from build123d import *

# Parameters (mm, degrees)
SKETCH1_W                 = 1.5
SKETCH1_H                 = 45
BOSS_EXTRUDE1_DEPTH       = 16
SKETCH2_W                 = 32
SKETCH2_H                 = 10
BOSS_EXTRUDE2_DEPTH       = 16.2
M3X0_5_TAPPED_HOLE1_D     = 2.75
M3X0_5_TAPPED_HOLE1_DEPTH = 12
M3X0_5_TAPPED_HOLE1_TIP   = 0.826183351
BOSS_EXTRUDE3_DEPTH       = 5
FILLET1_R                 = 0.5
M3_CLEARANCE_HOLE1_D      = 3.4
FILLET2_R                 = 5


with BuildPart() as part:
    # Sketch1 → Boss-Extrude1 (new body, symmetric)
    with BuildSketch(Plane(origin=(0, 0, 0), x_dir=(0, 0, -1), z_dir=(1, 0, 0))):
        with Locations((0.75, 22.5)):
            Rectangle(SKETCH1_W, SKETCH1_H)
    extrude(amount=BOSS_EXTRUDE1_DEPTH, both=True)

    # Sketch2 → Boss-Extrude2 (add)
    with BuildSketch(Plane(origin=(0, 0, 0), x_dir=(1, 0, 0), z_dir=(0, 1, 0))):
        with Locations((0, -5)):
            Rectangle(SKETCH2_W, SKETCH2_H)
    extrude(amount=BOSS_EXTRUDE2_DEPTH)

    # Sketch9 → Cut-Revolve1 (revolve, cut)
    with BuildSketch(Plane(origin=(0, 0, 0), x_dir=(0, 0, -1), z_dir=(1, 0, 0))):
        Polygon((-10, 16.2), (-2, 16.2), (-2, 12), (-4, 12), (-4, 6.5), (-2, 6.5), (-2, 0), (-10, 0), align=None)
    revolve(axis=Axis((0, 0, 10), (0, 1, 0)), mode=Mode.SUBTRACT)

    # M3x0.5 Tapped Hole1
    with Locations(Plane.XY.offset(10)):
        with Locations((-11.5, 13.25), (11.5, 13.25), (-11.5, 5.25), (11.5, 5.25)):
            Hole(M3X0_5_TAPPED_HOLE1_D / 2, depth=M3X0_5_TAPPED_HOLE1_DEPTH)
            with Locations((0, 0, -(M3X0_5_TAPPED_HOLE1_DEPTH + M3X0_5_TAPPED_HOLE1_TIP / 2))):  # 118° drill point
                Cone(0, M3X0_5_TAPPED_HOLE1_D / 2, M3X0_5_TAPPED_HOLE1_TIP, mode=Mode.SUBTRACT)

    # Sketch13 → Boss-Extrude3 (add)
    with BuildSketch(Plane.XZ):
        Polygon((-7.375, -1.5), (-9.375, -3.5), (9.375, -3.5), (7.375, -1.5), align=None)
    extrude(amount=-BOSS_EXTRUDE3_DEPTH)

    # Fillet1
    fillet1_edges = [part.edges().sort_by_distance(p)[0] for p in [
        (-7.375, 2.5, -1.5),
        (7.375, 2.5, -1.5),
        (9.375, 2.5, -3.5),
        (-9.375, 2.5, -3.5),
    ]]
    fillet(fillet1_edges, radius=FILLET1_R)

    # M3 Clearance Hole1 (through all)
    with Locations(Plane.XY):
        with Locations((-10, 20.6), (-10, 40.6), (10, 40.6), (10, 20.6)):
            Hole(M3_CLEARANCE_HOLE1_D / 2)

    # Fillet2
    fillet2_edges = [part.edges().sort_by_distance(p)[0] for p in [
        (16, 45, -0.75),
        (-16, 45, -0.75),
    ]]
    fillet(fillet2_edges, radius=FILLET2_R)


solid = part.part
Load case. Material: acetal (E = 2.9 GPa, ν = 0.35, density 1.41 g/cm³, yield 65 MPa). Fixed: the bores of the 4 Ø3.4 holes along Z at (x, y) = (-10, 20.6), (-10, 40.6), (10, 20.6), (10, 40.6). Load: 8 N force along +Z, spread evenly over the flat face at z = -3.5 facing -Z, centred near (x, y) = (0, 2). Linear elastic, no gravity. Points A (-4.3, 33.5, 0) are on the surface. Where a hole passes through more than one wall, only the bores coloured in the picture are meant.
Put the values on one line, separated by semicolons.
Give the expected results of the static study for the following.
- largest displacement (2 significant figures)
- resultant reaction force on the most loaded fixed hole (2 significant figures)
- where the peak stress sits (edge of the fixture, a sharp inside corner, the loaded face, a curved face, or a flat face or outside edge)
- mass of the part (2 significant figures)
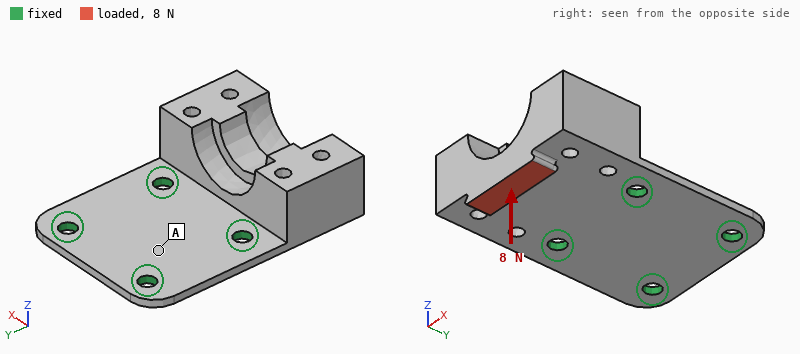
0.42 mm; 4.5 N; a flat face or outside edge; 8.2 g
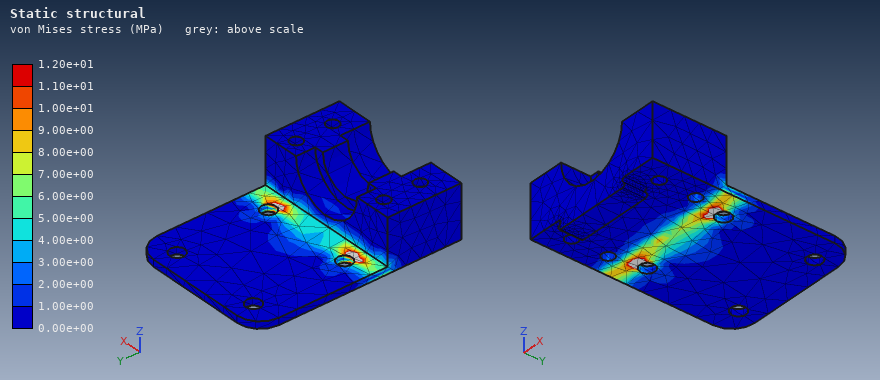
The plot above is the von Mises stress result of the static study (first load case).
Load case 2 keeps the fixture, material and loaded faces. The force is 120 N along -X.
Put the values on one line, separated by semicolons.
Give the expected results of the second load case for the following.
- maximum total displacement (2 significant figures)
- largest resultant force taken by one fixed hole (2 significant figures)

0.15 mm; 110 N
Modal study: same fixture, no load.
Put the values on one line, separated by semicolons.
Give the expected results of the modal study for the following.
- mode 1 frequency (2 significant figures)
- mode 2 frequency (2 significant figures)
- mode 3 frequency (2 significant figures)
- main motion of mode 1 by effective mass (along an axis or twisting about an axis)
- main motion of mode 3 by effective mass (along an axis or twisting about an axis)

410 Hz; 1900 Hz; 3500 Hz; along Z; along X
